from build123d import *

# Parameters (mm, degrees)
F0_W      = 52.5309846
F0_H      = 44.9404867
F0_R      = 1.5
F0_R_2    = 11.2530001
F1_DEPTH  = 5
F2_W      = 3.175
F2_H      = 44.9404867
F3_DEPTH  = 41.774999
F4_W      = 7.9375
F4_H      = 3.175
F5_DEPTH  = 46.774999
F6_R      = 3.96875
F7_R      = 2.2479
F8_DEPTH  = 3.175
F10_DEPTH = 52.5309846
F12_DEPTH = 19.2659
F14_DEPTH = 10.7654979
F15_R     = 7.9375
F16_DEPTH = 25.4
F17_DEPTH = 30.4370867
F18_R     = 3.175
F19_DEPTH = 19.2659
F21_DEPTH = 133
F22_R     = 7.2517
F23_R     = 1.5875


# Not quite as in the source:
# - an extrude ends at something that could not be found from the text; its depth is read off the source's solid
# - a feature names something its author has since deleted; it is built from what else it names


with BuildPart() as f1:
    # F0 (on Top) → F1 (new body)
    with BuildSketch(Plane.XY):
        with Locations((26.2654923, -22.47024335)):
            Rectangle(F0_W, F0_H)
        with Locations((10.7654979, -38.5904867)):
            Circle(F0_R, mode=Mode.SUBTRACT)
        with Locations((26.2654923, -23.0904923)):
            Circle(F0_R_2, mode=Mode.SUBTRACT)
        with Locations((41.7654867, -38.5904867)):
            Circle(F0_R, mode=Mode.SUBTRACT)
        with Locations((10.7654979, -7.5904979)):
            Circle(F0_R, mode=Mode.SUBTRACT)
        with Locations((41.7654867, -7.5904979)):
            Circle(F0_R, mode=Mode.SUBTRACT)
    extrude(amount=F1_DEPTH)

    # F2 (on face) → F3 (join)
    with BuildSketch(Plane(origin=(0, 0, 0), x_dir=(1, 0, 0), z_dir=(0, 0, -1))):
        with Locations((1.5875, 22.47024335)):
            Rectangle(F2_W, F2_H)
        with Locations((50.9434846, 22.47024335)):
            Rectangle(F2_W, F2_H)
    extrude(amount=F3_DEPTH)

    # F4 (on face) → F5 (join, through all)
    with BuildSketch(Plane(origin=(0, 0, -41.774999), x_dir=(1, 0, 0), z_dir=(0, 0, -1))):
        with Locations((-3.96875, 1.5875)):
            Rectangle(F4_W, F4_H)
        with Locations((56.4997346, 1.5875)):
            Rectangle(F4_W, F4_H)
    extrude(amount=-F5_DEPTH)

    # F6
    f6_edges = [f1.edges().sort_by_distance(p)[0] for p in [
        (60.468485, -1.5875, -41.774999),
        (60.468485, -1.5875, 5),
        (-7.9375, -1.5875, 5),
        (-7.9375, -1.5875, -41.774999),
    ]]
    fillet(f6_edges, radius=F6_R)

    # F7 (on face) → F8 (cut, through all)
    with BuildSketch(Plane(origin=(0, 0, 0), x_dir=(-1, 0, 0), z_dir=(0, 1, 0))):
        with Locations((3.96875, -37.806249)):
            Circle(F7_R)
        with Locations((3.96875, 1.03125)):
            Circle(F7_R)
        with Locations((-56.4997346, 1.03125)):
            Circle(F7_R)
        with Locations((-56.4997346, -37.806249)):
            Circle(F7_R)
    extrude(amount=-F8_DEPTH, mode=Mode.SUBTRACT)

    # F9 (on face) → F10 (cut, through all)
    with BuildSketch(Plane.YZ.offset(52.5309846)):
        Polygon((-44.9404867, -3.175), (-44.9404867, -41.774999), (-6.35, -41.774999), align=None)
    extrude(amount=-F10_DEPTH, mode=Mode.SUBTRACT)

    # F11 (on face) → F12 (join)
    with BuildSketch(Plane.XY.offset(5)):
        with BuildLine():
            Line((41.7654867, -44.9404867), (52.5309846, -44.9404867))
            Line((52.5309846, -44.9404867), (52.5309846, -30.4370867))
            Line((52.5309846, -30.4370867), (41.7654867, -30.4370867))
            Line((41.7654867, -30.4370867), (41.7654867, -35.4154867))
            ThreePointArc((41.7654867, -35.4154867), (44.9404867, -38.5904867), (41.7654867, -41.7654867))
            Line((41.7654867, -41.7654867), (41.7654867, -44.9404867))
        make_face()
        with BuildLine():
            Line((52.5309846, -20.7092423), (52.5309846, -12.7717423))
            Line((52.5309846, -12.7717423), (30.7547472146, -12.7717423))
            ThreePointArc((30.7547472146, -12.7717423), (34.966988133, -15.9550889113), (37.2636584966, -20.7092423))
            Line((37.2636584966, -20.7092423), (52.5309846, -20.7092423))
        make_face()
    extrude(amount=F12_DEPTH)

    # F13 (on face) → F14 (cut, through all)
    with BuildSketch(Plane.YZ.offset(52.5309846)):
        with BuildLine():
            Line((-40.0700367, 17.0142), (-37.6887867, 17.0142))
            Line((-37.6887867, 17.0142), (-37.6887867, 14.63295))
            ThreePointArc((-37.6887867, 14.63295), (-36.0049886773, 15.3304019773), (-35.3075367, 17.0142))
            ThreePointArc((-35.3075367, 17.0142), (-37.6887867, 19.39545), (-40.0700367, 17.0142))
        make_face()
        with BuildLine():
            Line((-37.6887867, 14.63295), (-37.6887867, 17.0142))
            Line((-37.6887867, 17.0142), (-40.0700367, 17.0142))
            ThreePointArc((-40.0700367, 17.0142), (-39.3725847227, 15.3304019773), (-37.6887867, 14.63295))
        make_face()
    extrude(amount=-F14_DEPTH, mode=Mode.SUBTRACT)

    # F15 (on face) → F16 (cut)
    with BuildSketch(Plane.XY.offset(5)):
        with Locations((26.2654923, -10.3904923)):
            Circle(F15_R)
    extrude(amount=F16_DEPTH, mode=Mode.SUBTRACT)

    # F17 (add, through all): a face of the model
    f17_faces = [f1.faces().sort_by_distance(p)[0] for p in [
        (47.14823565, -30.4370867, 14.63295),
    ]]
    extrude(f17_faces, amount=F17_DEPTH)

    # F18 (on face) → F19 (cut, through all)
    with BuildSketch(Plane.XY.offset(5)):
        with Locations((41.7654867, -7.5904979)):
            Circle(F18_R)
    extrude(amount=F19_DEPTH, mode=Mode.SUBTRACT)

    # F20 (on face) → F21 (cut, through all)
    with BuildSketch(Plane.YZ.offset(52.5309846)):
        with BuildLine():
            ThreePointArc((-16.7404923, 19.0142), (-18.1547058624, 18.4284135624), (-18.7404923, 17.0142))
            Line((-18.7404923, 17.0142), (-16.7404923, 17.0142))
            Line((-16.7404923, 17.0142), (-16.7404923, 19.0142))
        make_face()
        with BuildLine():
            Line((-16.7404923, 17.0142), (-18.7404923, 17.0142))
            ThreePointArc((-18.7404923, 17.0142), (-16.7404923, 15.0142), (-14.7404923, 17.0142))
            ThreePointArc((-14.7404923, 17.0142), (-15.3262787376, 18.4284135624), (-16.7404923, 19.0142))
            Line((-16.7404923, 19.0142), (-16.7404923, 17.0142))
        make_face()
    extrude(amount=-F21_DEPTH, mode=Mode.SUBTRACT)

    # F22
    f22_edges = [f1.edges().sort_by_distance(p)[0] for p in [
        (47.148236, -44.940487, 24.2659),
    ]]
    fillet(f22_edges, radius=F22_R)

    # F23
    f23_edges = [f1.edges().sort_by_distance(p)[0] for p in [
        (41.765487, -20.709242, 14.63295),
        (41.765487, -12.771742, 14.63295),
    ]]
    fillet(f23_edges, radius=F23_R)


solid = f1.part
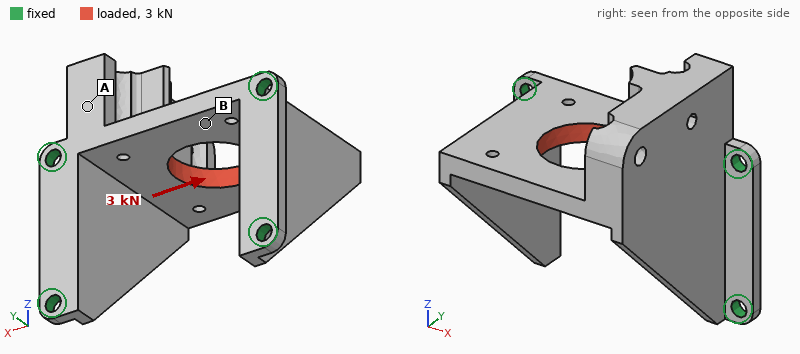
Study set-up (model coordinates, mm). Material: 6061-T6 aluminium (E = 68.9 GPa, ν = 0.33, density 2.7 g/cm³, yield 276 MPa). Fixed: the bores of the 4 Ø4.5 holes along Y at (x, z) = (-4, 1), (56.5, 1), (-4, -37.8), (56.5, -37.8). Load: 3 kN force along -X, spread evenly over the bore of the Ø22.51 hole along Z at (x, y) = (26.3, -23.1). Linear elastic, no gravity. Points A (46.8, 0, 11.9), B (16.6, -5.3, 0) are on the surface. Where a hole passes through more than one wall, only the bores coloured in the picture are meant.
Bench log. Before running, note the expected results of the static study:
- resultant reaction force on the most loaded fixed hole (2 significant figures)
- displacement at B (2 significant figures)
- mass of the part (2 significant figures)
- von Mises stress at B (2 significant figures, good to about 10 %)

1.9 kN
12 µm
76 g
25 MPa
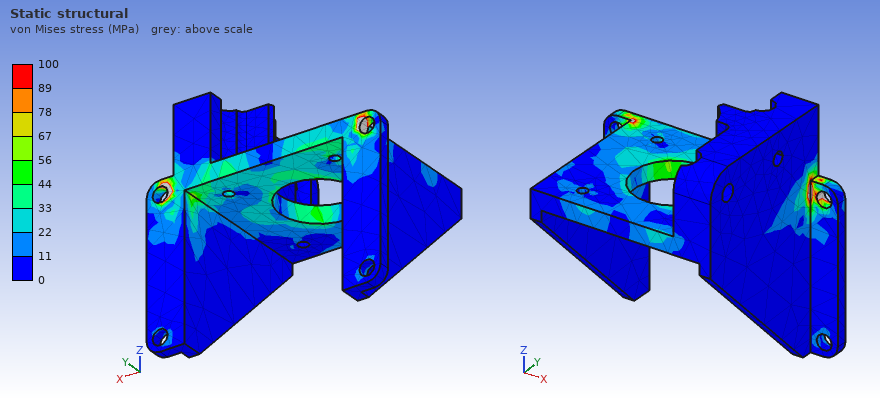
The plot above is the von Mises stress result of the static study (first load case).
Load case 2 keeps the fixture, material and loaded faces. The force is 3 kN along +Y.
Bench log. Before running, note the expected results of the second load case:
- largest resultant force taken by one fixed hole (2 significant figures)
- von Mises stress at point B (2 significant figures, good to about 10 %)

1.7 kN
11 MPa
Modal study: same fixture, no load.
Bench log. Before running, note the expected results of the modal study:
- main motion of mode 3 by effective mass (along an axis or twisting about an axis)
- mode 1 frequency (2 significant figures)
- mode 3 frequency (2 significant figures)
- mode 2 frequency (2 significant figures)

along X
3500 Hz
5900 Hz
4400 Hz
